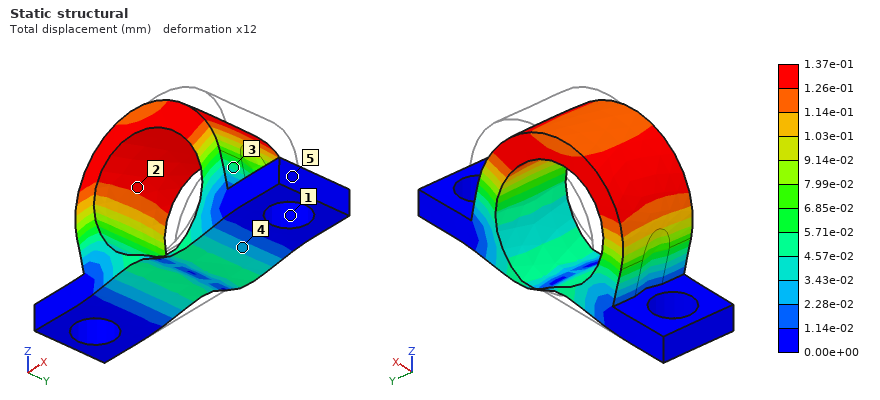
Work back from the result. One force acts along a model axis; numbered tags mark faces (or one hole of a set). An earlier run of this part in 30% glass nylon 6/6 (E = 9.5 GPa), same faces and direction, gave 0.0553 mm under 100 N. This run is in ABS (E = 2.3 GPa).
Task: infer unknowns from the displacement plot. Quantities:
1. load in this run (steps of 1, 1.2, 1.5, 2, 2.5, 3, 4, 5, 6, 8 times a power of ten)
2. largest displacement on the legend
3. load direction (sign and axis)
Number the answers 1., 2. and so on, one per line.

1. 60 N
2. 1.37e-01 mm
3. -X
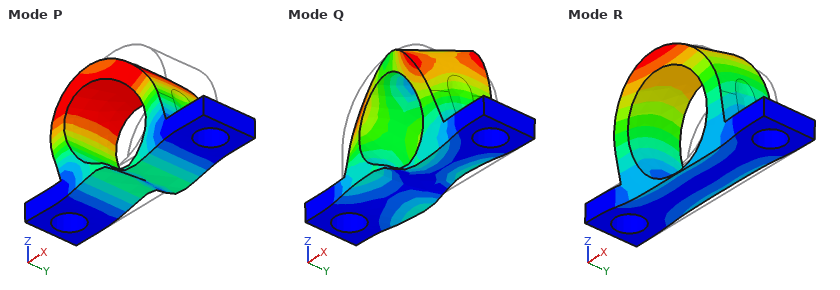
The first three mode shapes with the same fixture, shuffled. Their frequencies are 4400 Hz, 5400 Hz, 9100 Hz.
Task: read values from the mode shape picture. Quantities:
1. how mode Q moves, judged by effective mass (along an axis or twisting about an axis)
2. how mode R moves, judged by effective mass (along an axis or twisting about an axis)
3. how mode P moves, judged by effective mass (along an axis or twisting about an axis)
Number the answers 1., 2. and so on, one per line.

1. twisting about Z
2. along Y
3. along X
